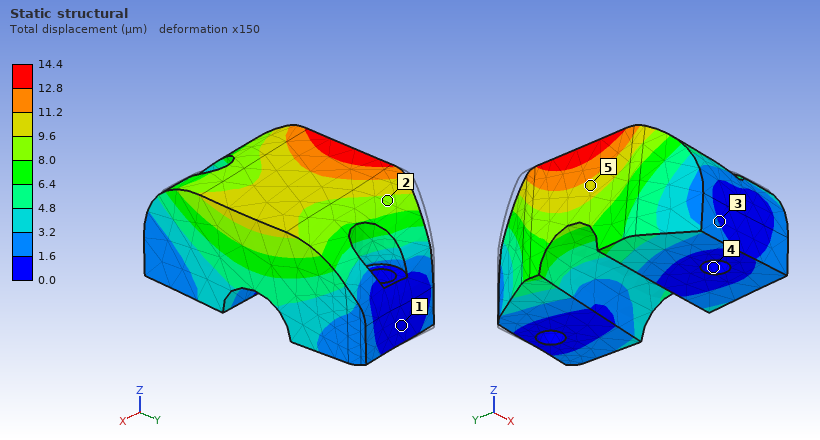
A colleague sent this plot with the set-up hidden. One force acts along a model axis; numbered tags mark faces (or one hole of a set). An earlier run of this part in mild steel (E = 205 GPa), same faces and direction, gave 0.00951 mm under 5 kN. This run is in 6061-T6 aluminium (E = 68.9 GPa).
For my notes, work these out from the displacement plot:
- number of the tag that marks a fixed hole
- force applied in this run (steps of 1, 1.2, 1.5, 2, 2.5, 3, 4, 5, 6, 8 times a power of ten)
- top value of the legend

4
2.5 kN
14.4 µm
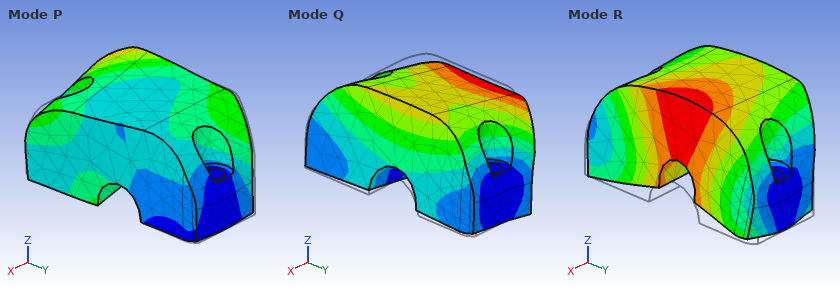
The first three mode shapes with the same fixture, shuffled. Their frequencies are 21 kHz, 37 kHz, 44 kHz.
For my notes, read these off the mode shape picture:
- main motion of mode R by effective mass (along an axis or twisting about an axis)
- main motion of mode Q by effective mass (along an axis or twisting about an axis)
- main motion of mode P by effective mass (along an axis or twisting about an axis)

along Z
along X
along Y
